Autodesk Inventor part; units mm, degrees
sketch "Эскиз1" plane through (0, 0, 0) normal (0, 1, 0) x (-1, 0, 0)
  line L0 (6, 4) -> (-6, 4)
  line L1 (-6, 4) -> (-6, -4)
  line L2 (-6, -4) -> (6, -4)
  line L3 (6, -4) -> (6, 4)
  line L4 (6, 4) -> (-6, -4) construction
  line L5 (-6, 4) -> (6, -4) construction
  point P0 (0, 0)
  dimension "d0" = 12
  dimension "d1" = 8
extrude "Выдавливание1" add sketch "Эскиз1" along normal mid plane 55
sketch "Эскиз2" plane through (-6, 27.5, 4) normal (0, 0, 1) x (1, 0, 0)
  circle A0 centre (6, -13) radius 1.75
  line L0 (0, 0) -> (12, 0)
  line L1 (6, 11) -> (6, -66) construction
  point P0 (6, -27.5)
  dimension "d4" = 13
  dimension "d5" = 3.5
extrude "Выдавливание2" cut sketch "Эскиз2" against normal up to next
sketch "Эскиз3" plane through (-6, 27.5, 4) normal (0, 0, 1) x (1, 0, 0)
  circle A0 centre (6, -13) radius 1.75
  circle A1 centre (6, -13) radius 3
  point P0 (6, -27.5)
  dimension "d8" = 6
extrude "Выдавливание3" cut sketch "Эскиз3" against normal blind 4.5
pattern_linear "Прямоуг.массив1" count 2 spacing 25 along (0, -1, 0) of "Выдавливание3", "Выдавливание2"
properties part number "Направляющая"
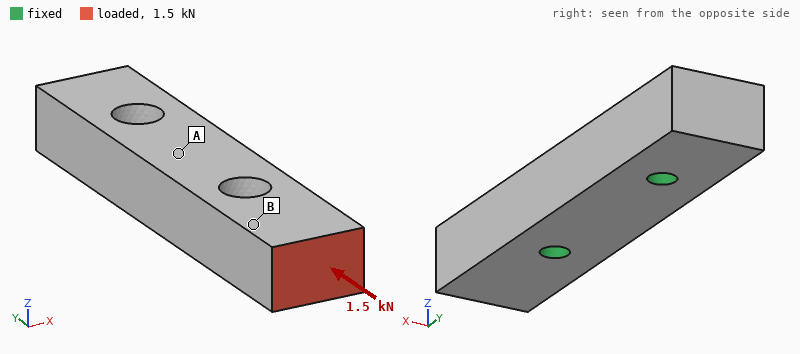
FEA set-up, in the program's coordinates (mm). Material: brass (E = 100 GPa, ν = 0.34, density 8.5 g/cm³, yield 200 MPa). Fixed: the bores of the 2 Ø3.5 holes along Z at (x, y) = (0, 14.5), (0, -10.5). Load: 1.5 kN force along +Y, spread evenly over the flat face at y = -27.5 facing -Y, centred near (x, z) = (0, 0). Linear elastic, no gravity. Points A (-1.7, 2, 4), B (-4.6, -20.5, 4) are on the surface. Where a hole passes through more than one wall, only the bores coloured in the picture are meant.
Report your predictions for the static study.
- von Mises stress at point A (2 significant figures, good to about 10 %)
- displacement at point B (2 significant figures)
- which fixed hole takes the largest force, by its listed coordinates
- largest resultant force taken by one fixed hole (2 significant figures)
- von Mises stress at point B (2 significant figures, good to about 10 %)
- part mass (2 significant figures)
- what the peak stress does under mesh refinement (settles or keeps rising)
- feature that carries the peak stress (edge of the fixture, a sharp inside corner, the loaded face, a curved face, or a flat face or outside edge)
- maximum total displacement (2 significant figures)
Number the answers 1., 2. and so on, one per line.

1. 6.5 MPa
2. 6.6 µm
3. (0, -10.5)
4. 1.2 kN
5. 16 MPa
6. 42 g
7. keeps rising
8. edge of the fixture
9. 9.6 µm
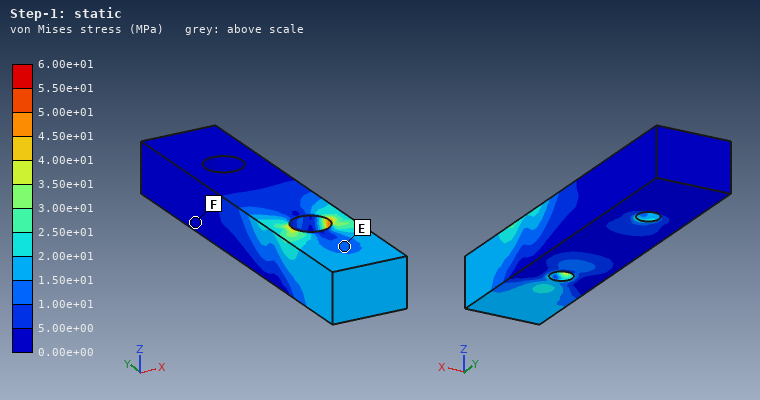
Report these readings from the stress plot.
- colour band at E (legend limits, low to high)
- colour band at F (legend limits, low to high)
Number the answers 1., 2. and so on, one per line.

1. 1.00e+01 to 1.50e+01 MPa
2. 0.00e+00 to 5.00e+00 MPa
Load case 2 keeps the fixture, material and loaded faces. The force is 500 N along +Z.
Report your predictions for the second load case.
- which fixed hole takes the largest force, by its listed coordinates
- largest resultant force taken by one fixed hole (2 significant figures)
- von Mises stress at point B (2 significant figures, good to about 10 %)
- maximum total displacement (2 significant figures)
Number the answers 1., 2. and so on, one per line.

1. (0, -10.5)
2. 850 N
3. 29 MPa
4. 36 µm
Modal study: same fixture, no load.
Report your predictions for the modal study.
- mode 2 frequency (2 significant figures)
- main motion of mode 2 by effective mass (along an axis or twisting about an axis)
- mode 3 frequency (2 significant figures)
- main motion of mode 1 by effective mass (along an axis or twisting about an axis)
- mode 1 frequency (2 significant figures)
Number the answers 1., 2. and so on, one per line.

1. 11 kHz
2. along X
3. 14 kHz
4. along Z
5. 9300 Hz
